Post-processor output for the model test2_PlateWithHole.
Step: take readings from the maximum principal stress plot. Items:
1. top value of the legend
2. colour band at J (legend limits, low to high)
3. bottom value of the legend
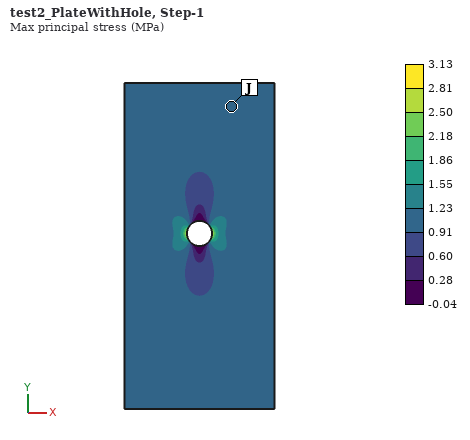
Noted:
3.13 MPa
0.91 to 1.23 MPa
-0.04 MPa
